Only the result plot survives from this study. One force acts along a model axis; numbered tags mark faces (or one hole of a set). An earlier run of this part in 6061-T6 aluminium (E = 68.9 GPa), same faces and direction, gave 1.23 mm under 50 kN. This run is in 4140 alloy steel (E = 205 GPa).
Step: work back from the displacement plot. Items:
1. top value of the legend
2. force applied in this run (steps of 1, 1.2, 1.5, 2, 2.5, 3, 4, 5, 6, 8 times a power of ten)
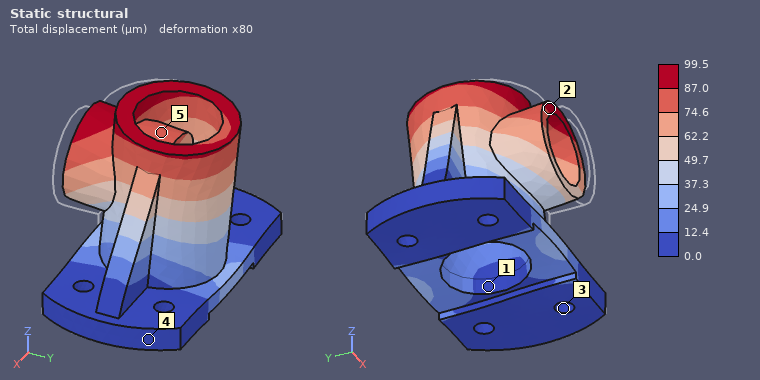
99.5 µm
12 kN
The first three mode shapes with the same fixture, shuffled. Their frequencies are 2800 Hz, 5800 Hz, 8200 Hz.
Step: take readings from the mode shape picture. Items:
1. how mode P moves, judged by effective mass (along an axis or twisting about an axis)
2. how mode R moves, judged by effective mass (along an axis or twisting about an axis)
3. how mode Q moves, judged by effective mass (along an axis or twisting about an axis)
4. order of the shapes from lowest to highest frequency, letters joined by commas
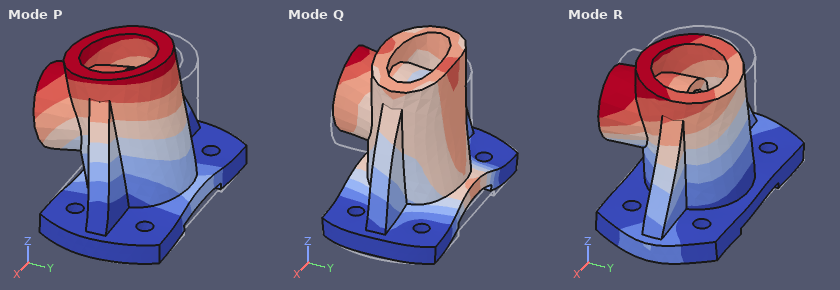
along Y
along X
along Z
P, R, Q
